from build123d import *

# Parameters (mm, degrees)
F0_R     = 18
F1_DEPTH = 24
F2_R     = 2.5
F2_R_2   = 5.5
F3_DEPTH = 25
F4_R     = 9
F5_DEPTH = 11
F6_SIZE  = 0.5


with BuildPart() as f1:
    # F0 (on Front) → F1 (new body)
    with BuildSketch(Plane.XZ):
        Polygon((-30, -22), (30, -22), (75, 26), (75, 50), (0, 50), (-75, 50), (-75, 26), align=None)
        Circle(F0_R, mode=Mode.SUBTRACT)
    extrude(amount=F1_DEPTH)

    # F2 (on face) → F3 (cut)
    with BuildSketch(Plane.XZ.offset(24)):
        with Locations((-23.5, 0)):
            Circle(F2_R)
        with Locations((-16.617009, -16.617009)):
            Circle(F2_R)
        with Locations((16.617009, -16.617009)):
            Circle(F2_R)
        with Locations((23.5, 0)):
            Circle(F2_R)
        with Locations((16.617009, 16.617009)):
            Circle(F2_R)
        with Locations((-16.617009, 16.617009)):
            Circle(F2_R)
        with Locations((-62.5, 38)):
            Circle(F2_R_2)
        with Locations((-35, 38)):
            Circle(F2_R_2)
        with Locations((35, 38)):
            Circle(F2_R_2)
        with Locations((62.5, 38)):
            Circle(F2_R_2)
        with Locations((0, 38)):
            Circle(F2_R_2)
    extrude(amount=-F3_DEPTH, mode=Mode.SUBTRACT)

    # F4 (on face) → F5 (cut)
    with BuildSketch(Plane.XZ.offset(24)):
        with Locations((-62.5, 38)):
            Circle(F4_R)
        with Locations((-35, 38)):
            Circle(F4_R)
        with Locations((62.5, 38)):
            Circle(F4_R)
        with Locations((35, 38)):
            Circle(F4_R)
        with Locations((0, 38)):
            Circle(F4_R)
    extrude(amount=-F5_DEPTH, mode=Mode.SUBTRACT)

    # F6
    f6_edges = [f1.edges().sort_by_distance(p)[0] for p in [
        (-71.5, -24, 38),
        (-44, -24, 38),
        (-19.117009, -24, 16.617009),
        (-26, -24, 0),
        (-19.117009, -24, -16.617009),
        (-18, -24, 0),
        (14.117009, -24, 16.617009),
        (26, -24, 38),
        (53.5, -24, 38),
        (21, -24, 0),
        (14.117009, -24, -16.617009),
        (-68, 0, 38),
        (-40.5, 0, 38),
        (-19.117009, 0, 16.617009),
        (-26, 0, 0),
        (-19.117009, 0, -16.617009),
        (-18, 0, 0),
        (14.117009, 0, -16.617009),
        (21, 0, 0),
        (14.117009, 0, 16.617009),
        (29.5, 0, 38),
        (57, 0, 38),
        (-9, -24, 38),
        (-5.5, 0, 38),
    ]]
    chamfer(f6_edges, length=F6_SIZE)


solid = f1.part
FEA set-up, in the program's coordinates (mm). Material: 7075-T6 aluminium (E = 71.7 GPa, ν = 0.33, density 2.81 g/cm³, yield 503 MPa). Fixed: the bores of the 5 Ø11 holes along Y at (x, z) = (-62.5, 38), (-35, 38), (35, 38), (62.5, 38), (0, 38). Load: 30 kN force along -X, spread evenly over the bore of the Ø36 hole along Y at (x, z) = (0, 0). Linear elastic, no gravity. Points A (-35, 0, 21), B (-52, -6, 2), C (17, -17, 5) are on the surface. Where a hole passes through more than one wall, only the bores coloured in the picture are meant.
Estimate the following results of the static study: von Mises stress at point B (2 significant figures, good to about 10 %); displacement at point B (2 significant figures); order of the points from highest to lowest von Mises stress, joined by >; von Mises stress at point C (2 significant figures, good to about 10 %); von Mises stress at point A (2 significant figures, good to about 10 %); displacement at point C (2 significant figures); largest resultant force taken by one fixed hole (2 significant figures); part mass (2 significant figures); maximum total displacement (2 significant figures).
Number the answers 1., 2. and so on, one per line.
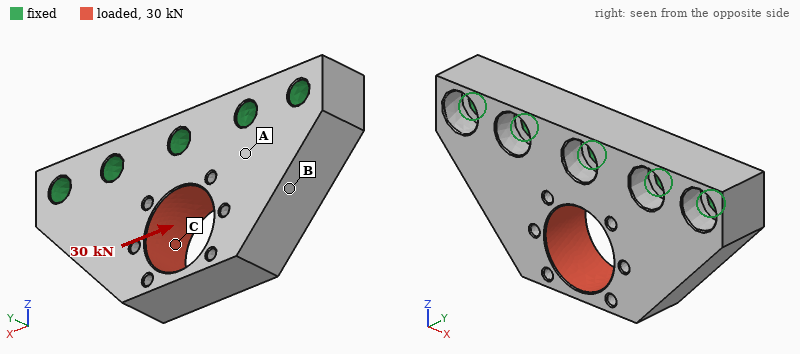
1. 31 MPa
2. 19 µm
3. C > B > A
4. 48 MPa
5. 13 MPa
6. 21 µm
7. 9.9 kN
8. 450 g
9. 52 µm
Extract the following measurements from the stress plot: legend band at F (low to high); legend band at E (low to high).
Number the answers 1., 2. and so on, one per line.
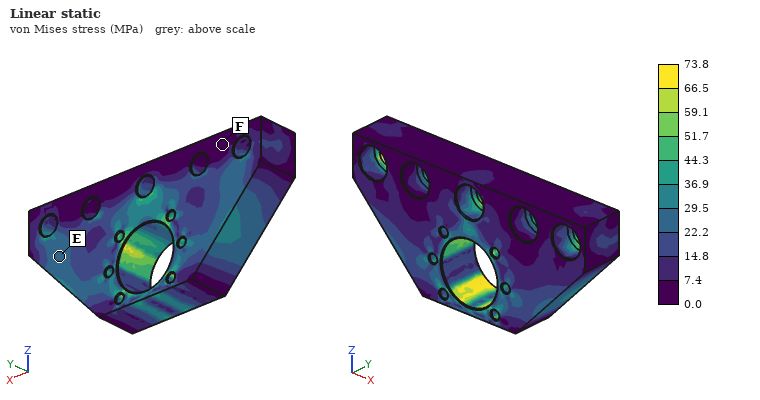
1. 0.0 to 7.4 MPa
2. 22.2 to 29.5 MPa
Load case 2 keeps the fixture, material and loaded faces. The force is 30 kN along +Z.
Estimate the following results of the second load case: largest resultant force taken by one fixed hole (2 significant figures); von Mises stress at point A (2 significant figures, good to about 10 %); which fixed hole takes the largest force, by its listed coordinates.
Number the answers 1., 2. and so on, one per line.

1. 9.8 kN
2. 13 MPa
3. (0, 38)
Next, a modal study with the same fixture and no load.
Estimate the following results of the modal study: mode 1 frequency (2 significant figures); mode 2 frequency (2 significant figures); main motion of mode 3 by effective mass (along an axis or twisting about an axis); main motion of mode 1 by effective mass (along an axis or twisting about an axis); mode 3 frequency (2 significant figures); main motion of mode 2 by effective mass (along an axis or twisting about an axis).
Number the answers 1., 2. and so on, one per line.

1. 4600 Hz
2. 7300 Hz
3. along X
4. along Y
5. 12 kHz
6. twisting about Z
